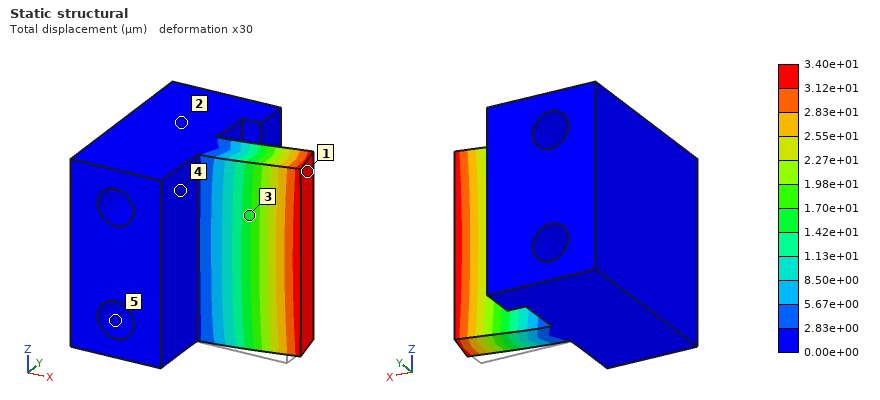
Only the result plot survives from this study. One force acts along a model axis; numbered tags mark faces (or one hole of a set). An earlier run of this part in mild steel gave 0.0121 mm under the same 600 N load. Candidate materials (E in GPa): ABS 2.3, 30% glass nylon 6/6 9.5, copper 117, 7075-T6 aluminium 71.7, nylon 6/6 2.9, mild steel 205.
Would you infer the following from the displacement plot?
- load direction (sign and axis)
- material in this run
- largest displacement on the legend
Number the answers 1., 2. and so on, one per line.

1. +Y
2. 7075-T6 aluminium
3. 3.40e+01 µm
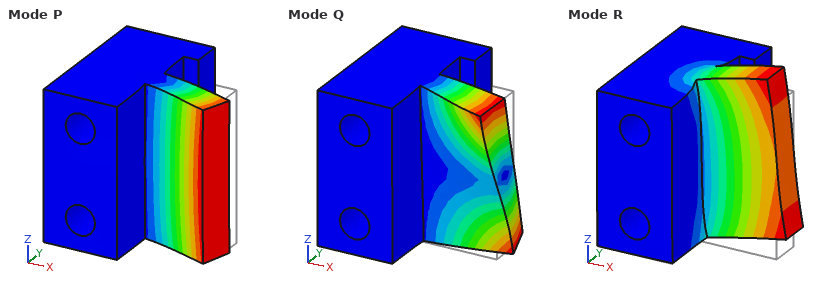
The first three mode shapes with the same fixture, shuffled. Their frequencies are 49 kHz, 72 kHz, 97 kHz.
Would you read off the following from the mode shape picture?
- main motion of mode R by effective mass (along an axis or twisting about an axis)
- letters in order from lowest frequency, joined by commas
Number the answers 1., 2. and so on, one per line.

1. along Z
2. P, Q, R
